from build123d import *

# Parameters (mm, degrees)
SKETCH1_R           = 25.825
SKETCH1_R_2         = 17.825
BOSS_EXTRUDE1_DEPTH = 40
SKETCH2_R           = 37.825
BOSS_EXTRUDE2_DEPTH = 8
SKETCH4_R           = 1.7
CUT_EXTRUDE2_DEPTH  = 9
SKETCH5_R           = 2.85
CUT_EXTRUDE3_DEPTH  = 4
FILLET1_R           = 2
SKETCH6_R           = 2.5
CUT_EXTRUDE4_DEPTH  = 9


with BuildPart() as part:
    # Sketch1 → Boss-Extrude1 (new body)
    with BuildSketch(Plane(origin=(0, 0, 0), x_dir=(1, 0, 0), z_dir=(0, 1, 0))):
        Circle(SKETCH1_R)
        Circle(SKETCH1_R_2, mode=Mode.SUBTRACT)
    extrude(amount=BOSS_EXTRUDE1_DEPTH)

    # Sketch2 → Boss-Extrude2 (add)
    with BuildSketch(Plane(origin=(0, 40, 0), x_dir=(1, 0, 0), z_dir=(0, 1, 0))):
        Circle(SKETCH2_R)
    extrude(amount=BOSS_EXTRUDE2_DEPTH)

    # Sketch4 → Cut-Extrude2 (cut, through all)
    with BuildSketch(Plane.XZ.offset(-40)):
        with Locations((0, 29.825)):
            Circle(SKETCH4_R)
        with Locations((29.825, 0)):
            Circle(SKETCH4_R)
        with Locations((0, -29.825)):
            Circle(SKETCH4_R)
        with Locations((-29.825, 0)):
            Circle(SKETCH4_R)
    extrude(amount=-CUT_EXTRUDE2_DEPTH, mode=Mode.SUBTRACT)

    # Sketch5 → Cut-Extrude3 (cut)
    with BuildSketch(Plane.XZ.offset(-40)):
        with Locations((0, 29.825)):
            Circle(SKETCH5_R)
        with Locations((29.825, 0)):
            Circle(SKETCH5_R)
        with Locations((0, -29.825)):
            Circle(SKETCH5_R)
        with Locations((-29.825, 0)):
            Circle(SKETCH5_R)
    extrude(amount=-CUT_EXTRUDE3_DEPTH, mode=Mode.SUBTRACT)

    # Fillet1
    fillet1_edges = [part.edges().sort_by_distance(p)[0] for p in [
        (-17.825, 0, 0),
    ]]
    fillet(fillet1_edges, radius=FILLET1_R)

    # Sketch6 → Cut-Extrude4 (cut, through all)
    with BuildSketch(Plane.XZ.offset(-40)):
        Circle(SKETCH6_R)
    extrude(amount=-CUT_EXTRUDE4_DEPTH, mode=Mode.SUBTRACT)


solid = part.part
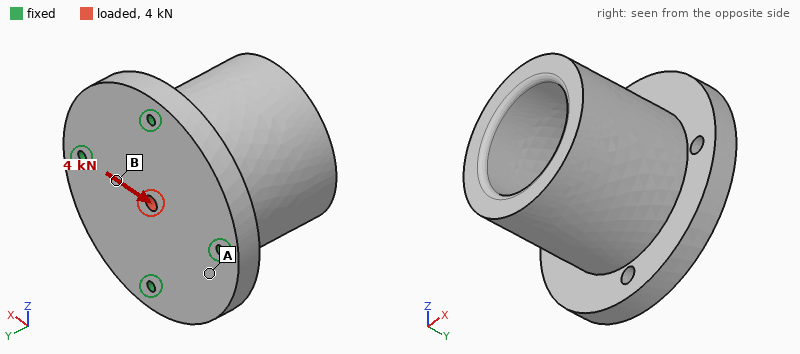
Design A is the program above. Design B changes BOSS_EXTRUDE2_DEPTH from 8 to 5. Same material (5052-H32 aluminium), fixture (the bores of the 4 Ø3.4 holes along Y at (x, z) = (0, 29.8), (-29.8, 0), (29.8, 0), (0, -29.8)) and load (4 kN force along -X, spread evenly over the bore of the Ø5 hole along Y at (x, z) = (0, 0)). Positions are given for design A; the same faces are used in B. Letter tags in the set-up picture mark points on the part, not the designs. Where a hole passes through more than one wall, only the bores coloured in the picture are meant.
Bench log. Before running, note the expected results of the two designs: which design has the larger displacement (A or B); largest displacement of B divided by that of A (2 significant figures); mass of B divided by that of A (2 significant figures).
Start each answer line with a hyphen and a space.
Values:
- B
- 1.9
- 0.83
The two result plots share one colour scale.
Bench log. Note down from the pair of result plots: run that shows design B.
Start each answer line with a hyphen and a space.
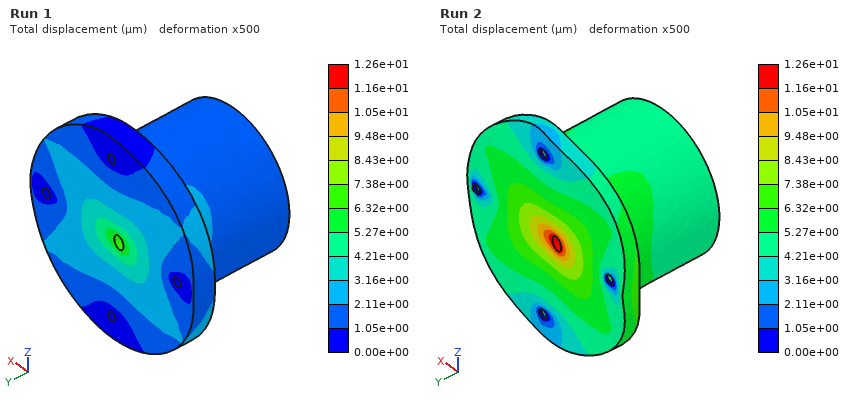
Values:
- Run 2
